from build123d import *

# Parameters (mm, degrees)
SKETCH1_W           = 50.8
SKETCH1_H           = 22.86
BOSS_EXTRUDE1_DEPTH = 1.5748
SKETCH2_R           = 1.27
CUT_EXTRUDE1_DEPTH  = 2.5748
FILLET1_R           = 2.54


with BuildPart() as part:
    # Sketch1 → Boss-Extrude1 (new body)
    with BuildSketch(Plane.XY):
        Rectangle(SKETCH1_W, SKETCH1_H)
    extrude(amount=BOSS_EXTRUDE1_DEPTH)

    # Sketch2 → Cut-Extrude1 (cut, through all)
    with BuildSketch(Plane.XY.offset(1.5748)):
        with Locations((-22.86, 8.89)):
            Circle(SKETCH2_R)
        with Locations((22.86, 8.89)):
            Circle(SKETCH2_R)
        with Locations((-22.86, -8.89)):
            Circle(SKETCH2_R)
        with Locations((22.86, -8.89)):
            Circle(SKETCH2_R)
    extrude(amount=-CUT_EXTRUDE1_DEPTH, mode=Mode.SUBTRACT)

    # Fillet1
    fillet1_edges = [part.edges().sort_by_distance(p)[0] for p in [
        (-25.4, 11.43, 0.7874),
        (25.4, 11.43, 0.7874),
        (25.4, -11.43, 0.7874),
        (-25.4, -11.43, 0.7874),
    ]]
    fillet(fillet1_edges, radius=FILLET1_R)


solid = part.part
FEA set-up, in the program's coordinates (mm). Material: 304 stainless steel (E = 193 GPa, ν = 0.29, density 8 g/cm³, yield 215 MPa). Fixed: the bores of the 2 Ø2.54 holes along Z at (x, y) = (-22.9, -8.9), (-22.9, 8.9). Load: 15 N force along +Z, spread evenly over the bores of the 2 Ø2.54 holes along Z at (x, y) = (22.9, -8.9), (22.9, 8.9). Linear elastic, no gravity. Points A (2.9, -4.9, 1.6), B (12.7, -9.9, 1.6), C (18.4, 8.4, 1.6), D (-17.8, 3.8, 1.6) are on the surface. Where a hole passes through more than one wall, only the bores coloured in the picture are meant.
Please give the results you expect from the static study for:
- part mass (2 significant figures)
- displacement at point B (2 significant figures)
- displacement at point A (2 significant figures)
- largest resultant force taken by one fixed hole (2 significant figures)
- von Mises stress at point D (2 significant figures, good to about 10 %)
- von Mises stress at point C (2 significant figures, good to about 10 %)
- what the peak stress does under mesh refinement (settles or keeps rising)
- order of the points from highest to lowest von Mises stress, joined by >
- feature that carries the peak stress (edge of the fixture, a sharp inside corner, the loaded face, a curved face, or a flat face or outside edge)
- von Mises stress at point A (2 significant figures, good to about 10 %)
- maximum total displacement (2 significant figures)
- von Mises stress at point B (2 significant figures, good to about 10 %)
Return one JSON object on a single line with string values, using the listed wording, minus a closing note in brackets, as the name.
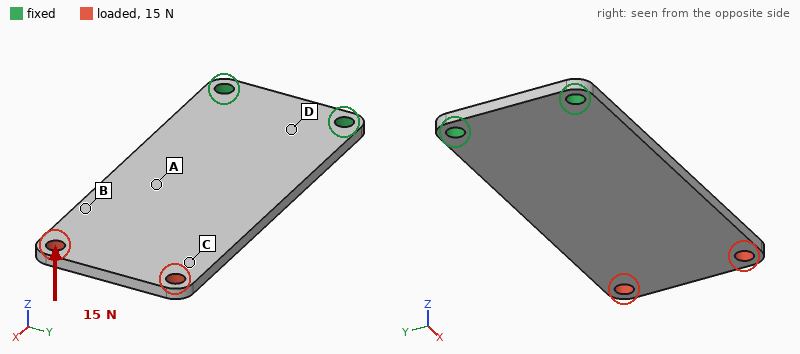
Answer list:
{"part mass": "14 g", "displacement at point B": "0.23 mm", "displacement at point A": "0.13 mm", "largest resultant force taken by one fixed hole": "7.5 N", "von Mises stress at point D": "57 MPa", "von Mises stress at point C": "9.0 MPa", "what the peak stress does under mesh refinement": "keeps rising", "order of the points from highest to lowest von Mises stress, joined by >": "D > A > B > C", "feature that carries the peak stress": "edge of the fixture", "von Mises stress at point A": "32 MPa", "maximum total displacement": "0.37 mm", "von Mises stress at point B": "17 MPa"}
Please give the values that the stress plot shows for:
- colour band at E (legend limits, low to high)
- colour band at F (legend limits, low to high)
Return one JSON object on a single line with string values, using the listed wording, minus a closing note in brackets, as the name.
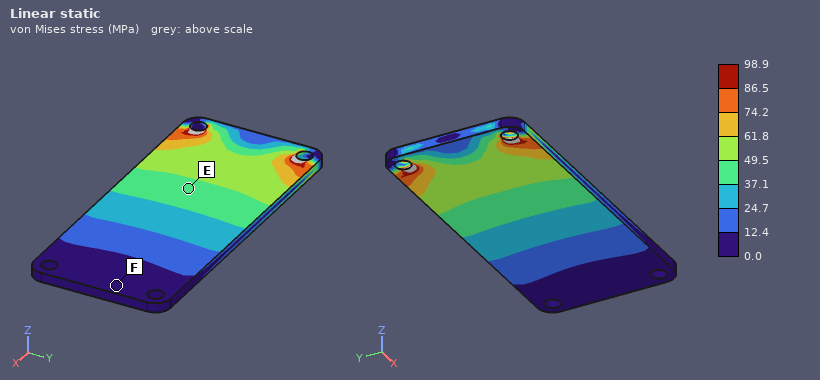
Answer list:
{"colour band at E": "37.1 to 49.5 MPa", "colour band at F": "0.0 to 12.4 MPa"}
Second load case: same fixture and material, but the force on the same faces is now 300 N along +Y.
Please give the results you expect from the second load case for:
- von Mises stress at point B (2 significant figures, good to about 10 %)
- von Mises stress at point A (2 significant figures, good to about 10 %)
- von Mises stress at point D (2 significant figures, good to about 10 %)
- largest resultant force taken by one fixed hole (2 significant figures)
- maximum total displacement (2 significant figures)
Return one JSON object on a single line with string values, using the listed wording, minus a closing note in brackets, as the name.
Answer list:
{"von Mises stress at point B": "20 MPa", "von Mises stress at point A": "26 MPa", "von Mises stress at point D": "26 MPa", "largest resultant force taken by one fixed hole": "760 N", "maximum total displacement": "42 µm"}
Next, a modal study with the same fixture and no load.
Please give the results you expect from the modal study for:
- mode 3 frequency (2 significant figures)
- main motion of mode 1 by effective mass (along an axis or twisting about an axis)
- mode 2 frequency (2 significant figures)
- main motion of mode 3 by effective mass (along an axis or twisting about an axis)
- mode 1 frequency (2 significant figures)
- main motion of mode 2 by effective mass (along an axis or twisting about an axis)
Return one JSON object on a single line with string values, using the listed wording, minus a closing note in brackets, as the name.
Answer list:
{"mode 3 frequency": "3400 Hz", "main motion of mode 1 by effective mass": "along Z", "mode 2 frequency": "2500 Hz", "main motion of mode 3 by effective mass": "along Z", "mode 1 frequency": "540 Hz", "main motion of mode 2 by effective mass": "twisting about X"}
